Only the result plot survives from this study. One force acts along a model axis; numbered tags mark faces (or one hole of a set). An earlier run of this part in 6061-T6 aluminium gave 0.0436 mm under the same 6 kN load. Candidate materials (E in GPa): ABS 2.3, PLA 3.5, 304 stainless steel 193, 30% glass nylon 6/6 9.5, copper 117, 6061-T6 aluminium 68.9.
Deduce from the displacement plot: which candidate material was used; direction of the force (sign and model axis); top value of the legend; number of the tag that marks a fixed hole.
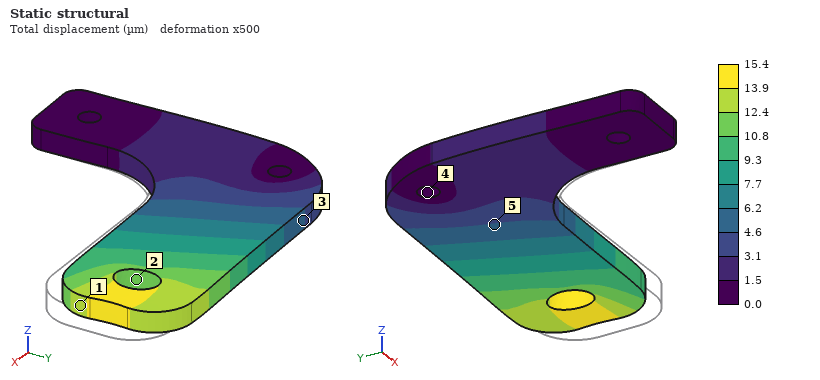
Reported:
304 stainless steel
-X
15.4 µm
4
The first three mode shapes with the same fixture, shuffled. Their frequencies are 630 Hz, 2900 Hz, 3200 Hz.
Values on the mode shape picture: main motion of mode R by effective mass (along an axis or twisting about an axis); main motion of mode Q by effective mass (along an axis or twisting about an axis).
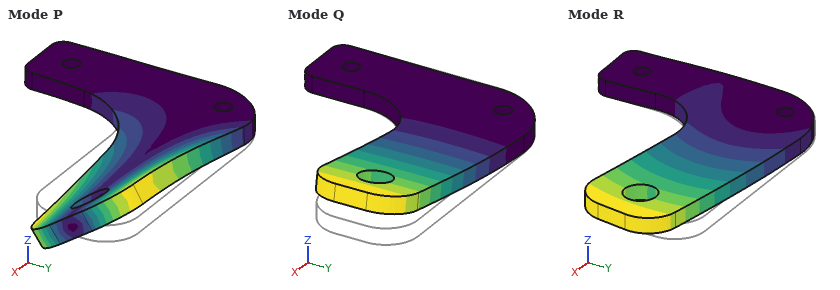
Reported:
along Y
along Z
